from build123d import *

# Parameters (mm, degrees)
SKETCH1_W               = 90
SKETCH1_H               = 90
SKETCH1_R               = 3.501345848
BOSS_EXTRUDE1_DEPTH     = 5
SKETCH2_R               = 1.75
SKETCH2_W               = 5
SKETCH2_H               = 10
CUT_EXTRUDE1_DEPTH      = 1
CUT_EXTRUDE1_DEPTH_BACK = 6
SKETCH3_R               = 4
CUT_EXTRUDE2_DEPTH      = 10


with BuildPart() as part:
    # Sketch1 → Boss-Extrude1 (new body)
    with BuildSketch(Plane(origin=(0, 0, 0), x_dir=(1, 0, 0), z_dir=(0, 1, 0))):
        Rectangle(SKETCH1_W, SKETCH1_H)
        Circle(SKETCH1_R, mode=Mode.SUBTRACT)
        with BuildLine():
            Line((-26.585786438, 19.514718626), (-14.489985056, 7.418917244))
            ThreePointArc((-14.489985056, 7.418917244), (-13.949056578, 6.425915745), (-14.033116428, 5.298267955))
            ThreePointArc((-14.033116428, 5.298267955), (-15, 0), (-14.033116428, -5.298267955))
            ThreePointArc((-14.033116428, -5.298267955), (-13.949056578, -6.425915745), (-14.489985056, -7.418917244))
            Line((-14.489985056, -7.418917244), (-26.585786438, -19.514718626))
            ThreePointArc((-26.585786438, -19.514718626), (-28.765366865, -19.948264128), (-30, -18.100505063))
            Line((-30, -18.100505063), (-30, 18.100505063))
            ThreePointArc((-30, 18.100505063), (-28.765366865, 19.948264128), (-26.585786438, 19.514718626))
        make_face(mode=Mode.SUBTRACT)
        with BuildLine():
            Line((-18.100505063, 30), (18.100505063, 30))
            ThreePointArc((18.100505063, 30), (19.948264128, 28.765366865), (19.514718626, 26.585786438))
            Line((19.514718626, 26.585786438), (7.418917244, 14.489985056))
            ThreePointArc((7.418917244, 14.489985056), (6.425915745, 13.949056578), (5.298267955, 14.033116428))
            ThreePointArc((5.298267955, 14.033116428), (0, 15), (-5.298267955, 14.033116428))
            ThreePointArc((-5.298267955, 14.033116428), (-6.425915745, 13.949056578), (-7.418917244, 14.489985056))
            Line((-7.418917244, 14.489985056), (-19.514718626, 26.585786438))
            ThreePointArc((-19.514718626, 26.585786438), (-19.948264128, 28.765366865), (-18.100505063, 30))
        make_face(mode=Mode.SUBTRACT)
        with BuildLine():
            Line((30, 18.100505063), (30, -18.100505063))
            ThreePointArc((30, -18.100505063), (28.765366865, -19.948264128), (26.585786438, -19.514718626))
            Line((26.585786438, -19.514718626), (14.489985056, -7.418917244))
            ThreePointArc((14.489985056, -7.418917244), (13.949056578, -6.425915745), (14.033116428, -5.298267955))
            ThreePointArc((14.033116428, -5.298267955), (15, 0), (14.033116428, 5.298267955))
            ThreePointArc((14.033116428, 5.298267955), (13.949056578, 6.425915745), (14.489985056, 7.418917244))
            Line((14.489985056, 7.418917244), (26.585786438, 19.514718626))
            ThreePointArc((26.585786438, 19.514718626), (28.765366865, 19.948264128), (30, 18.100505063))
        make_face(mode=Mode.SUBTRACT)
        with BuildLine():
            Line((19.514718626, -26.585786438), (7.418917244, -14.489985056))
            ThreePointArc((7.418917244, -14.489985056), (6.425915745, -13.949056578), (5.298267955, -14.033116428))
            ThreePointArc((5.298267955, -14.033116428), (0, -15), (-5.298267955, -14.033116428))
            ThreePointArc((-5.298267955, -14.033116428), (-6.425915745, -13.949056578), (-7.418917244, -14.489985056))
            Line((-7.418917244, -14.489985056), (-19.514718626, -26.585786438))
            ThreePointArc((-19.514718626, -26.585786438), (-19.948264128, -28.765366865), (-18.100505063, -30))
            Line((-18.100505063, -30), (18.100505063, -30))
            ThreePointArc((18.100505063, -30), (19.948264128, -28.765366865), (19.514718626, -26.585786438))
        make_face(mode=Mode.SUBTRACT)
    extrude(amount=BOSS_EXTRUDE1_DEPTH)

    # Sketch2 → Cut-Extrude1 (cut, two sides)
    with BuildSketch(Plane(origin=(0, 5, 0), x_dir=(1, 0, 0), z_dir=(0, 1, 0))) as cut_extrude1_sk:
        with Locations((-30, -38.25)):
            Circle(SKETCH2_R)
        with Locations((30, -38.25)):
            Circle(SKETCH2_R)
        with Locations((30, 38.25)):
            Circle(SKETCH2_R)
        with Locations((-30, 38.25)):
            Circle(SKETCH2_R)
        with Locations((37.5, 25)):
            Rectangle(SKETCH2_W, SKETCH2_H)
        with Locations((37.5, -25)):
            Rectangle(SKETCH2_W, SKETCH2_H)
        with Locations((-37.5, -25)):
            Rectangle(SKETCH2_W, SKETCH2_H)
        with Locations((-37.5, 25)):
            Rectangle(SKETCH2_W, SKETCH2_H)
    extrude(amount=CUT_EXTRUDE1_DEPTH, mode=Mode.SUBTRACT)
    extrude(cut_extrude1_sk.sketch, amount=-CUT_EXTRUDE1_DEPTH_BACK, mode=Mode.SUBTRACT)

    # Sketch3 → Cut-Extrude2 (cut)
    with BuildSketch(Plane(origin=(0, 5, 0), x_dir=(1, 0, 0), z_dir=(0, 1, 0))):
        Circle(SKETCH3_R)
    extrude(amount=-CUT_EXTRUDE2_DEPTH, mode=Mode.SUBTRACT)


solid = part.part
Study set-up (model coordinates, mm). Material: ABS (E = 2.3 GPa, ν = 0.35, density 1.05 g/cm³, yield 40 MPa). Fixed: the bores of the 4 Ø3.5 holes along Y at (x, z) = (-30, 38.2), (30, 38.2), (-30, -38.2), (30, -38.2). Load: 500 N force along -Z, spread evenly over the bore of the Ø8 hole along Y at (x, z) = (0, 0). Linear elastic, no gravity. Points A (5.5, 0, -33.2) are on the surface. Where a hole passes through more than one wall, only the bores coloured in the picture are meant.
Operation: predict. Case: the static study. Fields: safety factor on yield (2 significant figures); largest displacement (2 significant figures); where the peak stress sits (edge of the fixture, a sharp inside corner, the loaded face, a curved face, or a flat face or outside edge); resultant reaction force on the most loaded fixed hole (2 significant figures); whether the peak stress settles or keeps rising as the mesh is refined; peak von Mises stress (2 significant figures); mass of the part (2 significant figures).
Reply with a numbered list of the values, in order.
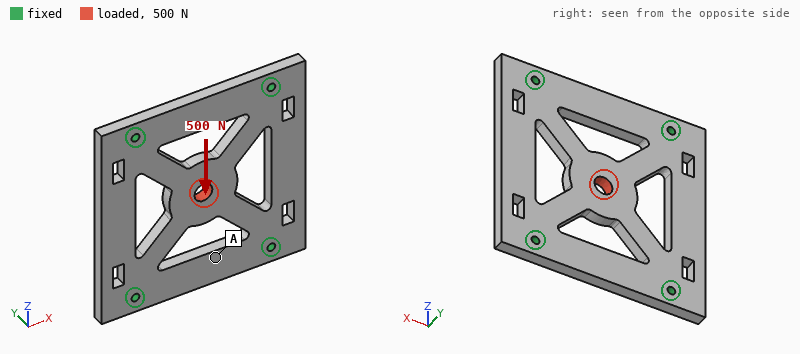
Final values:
1. 3.7
2. 86 µm
3. a curved face
4. 140 N
5. settles
6. 11 MPa
7. 31 g
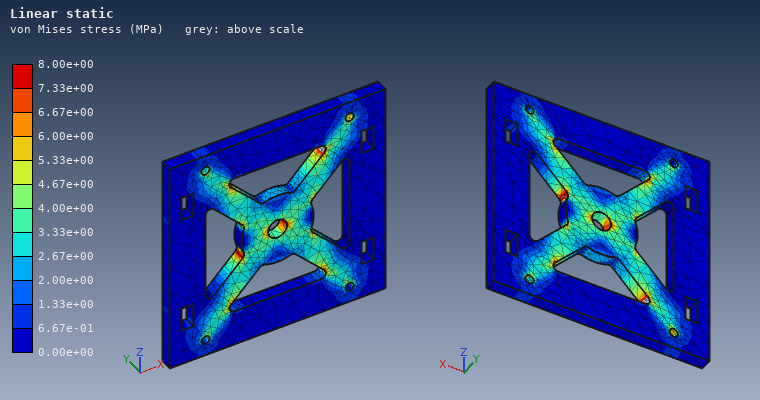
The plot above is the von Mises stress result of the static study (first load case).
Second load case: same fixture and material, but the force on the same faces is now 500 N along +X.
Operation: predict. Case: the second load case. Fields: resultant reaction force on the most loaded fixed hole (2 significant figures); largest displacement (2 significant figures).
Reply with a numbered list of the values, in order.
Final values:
1. 150 N
2. 0.10 mm
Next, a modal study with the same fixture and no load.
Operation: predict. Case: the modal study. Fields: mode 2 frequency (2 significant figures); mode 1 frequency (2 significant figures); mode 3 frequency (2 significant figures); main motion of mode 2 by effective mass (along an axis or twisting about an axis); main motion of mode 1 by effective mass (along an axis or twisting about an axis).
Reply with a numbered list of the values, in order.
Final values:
1. 1300 Hz
2. 980 Hz
3. 1300 Hz
4. twisting about Z
5. along Y
